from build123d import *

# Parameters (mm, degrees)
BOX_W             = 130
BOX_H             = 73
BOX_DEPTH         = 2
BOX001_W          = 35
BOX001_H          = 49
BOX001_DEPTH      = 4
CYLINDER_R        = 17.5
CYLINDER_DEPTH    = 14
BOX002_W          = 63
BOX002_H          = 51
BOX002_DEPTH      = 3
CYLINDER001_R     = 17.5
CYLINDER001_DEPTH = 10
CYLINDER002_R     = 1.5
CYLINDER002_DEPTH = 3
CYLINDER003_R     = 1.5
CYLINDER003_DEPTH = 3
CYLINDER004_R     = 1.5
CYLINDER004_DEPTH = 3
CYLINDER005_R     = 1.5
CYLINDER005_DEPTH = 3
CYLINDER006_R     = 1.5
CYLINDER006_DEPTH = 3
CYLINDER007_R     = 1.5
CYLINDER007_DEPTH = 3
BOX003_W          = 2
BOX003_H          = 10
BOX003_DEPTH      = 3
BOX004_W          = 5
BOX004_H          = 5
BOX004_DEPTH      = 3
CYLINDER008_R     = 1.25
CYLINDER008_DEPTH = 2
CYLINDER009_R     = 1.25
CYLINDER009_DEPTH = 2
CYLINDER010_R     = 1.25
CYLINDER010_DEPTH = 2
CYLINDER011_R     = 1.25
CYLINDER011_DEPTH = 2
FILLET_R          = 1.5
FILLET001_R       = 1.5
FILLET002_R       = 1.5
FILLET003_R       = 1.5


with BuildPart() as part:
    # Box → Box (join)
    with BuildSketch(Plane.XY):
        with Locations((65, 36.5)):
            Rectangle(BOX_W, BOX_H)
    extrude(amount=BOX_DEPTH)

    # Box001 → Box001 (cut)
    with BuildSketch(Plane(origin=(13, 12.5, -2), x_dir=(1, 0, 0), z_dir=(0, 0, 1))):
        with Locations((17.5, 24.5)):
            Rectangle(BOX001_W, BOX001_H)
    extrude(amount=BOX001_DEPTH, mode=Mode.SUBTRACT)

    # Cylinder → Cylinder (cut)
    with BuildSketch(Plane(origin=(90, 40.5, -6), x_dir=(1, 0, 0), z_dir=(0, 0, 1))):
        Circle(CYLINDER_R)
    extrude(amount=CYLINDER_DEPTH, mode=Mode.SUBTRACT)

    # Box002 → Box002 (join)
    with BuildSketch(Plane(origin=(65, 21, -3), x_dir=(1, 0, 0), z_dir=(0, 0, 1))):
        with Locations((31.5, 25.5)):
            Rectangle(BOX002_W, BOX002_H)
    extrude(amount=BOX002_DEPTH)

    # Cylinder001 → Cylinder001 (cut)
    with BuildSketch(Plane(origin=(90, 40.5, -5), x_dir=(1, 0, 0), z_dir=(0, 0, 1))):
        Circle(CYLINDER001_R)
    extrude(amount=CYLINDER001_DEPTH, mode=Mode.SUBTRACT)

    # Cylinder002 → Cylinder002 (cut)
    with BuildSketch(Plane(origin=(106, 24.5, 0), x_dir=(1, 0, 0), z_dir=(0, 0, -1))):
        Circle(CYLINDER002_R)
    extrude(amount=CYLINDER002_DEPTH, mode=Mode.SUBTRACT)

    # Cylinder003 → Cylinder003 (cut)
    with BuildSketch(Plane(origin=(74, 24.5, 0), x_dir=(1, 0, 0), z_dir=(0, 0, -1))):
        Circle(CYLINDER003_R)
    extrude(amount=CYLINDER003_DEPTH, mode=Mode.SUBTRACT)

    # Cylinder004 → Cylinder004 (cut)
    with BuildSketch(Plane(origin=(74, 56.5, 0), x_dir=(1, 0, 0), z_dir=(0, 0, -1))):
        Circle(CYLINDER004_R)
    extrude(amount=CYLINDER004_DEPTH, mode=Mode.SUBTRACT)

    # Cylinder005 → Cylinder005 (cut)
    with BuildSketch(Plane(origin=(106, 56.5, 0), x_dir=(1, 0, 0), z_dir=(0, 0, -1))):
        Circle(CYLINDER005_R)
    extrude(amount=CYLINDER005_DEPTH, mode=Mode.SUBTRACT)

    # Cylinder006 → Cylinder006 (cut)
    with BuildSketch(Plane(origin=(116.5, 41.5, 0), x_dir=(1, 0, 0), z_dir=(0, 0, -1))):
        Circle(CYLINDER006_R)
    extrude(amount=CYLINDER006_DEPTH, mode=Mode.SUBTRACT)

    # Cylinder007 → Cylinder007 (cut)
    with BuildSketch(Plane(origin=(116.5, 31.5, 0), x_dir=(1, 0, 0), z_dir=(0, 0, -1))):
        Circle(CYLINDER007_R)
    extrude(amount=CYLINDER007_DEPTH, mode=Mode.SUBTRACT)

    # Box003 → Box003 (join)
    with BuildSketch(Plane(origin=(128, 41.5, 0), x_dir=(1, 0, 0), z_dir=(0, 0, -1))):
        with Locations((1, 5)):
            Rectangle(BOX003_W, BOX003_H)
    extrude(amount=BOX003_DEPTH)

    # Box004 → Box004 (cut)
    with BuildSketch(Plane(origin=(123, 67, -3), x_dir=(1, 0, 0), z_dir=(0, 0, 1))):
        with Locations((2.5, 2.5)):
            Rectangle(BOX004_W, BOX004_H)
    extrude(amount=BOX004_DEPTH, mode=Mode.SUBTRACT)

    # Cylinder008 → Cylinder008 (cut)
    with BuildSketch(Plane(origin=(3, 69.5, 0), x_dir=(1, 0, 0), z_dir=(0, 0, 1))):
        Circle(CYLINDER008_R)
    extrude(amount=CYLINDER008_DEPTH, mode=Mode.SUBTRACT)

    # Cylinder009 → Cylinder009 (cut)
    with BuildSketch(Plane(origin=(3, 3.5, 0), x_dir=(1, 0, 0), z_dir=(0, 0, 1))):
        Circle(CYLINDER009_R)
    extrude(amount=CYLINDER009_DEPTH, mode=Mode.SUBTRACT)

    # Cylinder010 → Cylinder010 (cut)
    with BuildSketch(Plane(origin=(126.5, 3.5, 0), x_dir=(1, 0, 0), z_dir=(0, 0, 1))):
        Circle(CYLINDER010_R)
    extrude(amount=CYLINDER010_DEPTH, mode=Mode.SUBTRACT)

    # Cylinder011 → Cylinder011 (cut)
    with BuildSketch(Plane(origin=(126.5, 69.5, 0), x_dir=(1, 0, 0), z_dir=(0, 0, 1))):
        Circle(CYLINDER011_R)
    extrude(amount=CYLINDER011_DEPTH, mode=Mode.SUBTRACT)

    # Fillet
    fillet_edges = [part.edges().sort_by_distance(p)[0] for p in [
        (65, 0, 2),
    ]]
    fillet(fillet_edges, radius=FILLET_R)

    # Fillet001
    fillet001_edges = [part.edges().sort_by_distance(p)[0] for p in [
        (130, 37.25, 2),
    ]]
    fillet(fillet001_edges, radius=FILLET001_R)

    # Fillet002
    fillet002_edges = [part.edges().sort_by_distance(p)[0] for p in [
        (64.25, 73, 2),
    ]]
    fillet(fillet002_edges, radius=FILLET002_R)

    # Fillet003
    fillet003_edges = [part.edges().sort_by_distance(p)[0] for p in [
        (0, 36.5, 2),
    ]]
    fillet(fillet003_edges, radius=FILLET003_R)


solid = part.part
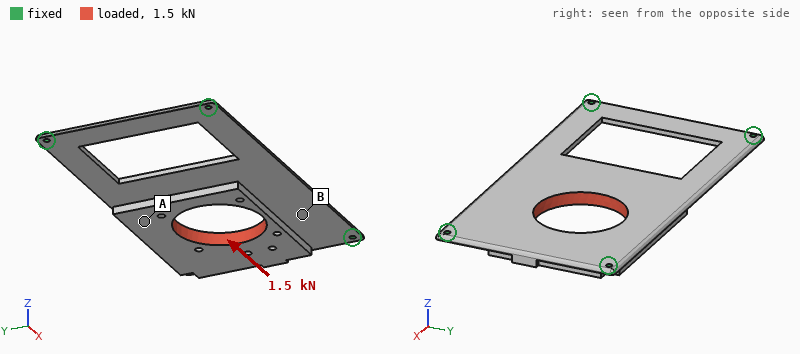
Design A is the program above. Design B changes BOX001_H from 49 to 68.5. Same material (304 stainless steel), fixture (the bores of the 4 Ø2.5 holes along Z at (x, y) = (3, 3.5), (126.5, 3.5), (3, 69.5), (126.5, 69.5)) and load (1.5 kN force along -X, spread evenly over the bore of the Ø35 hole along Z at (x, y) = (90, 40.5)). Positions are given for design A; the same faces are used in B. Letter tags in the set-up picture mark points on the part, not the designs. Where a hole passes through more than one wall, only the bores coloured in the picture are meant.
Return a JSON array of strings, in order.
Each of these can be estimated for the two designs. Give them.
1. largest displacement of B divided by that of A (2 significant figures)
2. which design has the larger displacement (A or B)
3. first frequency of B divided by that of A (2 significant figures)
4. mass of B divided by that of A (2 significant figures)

["1.9", "B", "0.76", "0.93"]
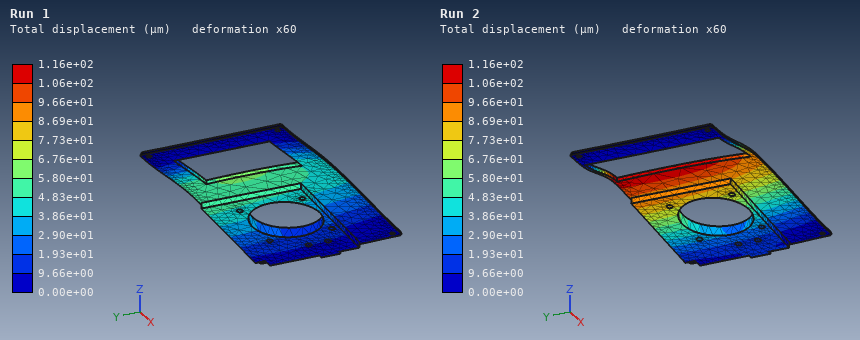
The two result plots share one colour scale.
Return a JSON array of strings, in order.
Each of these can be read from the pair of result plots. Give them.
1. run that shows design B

["Run 2"]
